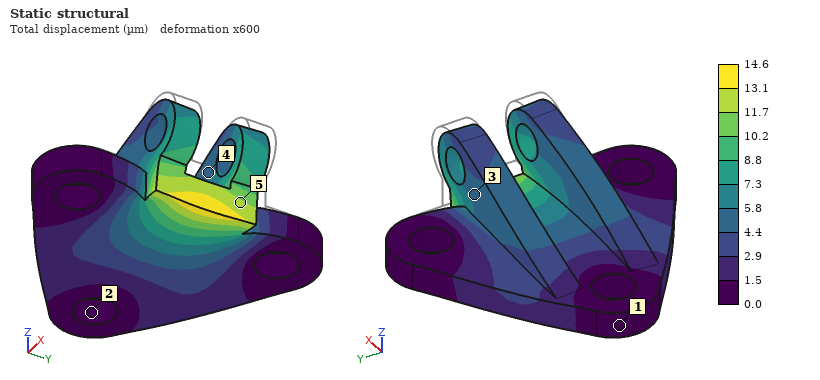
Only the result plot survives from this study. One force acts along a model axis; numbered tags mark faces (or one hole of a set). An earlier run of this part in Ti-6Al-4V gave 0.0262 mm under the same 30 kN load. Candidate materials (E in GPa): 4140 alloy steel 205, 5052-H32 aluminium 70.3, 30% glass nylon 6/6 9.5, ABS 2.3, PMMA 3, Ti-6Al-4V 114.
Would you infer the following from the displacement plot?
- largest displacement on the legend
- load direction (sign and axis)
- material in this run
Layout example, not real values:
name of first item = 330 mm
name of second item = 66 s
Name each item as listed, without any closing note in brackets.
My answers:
largest displacement on the legend = 14.6 µm
load direction = -X
material in this run = 4140 alloy steel
